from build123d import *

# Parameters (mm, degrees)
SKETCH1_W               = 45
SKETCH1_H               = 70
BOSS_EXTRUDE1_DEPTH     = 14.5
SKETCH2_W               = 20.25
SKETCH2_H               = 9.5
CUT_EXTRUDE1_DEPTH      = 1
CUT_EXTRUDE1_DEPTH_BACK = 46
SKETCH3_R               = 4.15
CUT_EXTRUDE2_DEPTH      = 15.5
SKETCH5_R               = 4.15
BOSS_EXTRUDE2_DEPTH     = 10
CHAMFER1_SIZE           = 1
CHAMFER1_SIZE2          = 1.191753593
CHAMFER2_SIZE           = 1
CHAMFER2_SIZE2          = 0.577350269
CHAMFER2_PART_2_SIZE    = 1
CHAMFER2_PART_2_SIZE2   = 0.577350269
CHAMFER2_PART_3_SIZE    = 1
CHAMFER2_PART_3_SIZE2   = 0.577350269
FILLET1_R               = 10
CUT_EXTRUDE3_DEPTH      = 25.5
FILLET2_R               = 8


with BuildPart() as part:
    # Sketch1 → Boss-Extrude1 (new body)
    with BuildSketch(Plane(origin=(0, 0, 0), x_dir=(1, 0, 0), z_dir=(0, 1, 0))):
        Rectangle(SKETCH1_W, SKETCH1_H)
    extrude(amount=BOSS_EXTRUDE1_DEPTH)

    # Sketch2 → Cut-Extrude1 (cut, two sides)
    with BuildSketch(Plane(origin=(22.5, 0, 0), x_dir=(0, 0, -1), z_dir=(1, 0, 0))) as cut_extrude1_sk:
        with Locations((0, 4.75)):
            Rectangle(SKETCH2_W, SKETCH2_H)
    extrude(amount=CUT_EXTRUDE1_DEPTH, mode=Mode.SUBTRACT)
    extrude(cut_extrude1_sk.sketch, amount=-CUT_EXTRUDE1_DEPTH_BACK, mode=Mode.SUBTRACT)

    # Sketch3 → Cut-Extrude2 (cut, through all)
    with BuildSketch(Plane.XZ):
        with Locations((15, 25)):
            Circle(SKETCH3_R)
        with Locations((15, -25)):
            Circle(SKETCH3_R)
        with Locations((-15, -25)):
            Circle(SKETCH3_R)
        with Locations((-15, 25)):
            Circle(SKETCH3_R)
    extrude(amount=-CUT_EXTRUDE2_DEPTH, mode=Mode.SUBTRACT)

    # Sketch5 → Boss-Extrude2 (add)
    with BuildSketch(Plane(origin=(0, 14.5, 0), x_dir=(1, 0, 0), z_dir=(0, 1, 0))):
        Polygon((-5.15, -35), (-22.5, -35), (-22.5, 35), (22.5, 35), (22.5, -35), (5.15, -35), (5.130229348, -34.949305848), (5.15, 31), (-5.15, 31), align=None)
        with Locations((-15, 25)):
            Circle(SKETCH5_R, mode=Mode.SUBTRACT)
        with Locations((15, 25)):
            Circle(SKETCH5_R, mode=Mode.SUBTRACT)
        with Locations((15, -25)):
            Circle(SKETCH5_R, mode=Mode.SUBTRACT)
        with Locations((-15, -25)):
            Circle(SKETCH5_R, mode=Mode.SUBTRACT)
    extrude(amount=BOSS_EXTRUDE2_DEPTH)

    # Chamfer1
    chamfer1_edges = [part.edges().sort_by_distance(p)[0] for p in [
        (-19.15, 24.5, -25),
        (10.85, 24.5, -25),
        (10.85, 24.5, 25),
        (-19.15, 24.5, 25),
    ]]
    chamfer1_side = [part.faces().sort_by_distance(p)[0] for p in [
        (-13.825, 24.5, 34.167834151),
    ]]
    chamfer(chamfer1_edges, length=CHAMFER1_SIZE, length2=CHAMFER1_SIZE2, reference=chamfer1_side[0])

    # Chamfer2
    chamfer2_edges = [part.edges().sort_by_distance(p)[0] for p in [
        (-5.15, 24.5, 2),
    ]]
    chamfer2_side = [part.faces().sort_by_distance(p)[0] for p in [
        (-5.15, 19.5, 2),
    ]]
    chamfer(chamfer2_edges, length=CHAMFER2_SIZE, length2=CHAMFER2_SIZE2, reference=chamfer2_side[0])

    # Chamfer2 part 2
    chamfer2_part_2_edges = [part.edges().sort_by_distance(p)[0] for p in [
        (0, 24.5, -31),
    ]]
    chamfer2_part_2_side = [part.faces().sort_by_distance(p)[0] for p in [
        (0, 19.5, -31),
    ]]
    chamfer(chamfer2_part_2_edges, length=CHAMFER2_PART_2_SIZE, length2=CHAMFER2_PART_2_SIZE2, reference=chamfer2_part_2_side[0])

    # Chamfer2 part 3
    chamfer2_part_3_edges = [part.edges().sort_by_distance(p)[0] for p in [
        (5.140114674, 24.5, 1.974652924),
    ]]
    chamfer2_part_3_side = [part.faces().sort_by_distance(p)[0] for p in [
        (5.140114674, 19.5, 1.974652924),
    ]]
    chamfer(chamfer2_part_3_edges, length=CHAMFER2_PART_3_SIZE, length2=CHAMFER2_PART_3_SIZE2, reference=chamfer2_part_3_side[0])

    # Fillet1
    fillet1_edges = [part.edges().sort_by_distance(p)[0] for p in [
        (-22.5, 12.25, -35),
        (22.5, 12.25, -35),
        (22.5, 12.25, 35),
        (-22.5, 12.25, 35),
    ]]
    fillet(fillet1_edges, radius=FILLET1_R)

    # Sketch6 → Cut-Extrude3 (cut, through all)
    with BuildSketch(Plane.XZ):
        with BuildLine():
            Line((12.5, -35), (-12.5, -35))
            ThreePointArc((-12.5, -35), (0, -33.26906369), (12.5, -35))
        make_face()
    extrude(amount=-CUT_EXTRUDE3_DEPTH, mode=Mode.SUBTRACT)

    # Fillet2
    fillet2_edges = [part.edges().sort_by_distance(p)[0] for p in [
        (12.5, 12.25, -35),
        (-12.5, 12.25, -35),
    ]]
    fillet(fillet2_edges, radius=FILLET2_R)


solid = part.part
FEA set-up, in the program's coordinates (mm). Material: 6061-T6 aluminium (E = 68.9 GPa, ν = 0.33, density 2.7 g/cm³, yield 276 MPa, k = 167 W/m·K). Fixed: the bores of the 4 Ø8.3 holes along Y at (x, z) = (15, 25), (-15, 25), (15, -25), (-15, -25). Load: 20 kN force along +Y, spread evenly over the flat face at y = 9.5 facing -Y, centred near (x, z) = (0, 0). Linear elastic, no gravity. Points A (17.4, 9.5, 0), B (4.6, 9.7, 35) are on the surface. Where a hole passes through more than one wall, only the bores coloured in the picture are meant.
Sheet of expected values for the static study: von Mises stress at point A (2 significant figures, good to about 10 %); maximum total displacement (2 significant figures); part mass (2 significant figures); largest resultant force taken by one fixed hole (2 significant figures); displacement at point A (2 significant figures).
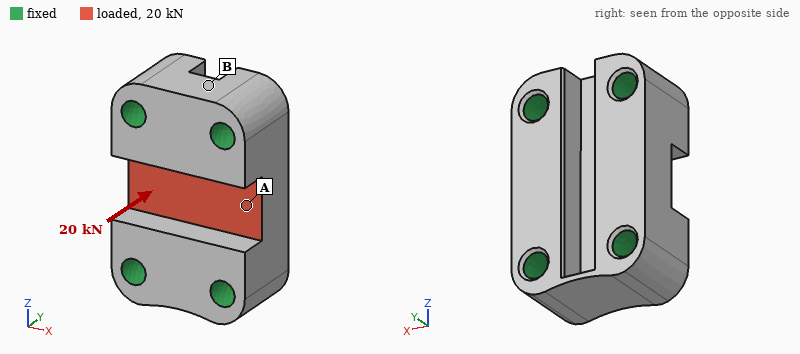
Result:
28 MPa
24 µm
140 g
5.1 kN
16 µm
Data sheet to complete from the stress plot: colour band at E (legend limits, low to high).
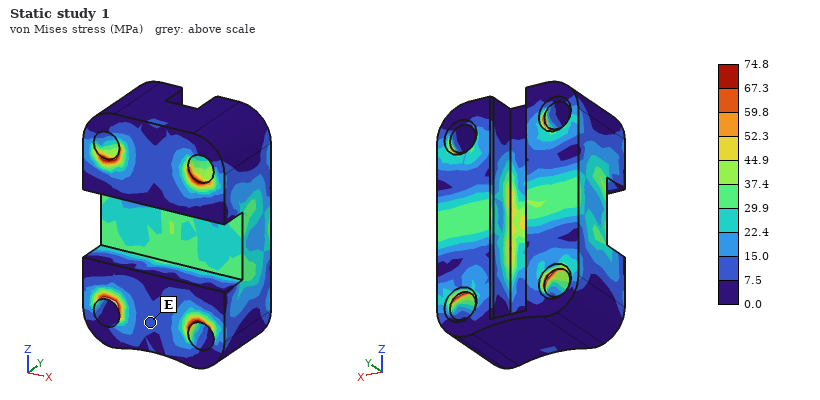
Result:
7.5 to 15.0 MPa
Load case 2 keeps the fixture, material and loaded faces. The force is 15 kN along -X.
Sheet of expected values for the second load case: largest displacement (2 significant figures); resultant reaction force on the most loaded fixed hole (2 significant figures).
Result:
19 µm
4.3 kN
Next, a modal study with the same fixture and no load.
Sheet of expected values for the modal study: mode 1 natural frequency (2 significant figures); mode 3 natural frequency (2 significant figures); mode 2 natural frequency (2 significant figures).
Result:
28 kHz
32 kHz
29 kHz
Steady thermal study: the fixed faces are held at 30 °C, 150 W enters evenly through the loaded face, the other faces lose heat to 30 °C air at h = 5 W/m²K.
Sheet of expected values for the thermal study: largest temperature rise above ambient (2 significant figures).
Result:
17 K
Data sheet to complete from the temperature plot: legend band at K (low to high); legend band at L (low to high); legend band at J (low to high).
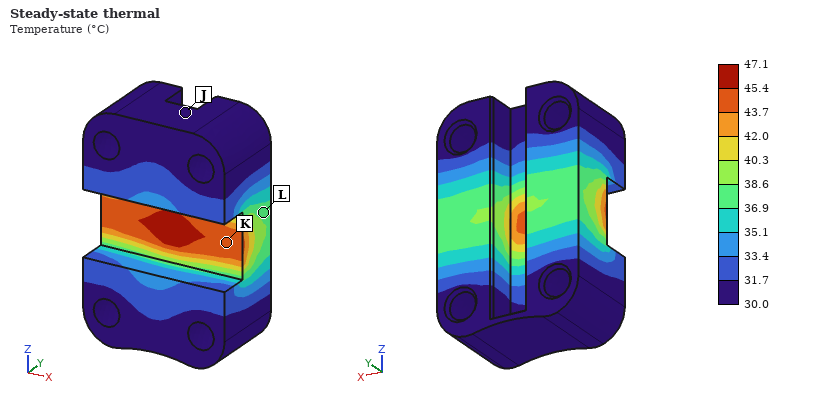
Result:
43.7 to 45.4 °C
36.9 to 38.6 °C
30.0 to 31.7 °C
